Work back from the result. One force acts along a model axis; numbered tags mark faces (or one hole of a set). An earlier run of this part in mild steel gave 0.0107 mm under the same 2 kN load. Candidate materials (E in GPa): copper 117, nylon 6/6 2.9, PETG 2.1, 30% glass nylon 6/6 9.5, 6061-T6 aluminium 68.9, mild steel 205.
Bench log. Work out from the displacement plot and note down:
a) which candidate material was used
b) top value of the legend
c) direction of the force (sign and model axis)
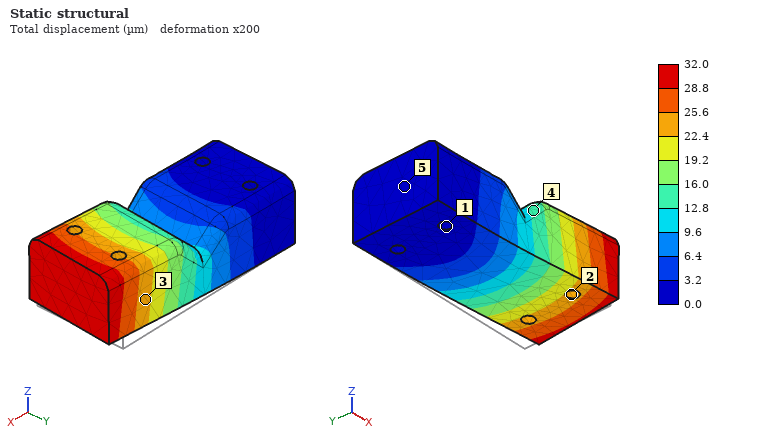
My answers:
6061-T6 aluminium
32.0 µm
-Y
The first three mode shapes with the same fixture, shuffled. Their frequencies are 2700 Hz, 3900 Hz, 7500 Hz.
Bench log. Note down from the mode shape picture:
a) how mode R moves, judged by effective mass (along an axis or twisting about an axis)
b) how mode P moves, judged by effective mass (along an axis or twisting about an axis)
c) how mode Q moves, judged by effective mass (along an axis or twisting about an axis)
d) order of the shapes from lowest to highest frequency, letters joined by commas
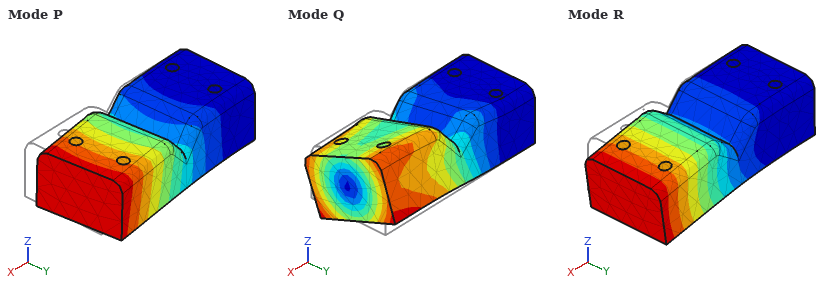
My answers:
along Z
along Y
twisting about X
R, P, Q
